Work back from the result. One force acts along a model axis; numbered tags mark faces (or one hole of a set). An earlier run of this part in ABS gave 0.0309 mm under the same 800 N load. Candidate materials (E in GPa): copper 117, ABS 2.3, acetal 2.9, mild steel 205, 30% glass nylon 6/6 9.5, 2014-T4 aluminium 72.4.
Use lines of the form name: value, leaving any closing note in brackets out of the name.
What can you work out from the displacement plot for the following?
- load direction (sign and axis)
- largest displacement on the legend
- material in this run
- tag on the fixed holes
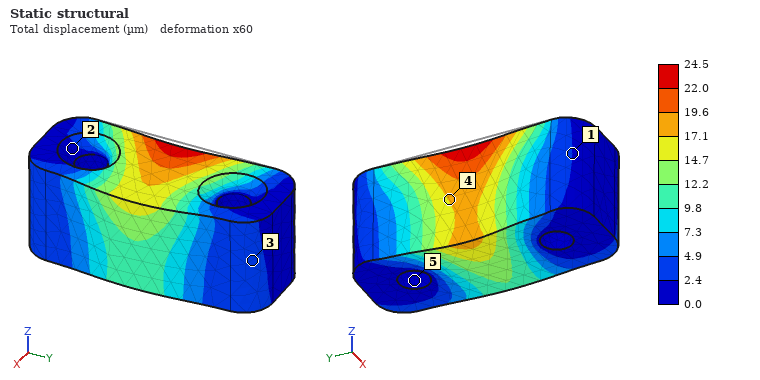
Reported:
load direction: +X
largest displacement on the legend: 24.5 µm
material in this run: acetal
tag on the fixed holes: 5
